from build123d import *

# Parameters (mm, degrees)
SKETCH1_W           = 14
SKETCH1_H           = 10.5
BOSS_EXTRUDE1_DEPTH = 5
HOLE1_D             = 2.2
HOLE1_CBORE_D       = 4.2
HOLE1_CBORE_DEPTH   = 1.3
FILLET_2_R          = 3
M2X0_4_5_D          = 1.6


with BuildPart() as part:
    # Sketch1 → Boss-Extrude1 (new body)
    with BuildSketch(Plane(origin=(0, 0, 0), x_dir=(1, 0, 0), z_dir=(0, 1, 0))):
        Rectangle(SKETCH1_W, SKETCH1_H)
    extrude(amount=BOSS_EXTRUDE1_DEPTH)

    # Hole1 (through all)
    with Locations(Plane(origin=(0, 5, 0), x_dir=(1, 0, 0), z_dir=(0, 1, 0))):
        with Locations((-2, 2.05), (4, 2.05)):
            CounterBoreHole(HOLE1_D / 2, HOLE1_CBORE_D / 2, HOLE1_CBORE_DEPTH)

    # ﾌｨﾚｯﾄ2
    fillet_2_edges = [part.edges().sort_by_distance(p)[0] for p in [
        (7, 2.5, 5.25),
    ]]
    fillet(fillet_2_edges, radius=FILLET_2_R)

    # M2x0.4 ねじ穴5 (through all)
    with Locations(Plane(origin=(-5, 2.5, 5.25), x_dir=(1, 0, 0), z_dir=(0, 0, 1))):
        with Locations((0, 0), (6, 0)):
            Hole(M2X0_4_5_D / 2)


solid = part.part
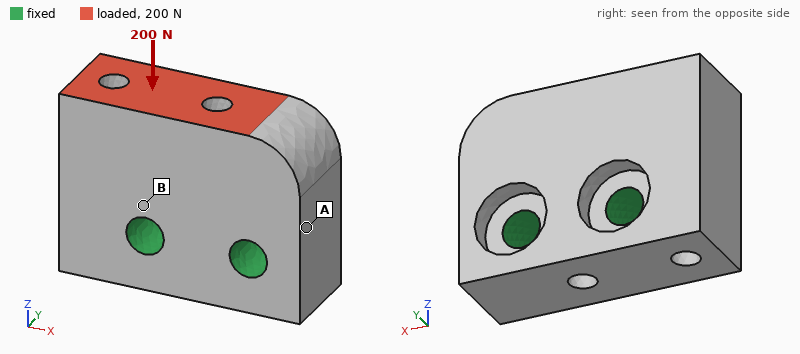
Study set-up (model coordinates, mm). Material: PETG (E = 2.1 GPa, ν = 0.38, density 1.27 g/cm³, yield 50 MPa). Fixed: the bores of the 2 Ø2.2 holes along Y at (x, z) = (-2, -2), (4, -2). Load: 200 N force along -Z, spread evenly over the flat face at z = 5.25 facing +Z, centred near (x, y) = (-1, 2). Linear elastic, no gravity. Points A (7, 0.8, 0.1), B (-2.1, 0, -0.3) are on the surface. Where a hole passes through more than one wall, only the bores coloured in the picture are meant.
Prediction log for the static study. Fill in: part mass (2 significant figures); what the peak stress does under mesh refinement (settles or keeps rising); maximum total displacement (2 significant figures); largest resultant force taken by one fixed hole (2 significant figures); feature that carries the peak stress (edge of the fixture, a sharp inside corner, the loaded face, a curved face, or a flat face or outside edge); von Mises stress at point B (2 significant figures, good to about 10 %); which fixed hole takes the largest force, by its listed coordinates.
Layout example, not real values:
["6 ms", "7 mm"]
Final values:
["0.79 g", "keeps rising", "45 µm", "160 N", "edge of the fixture", "5.7 MPa", "(-2, -2)"]
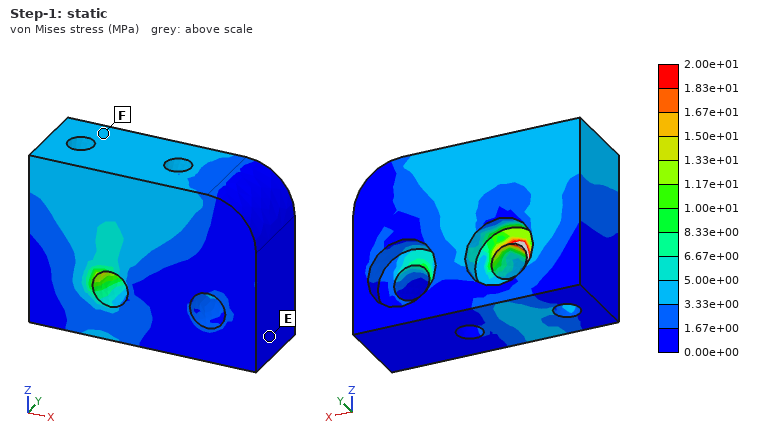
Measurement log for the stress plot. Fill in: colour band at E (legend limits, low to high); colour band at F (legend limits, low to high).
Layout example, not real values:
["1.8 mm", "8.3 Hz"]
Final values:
["0.00e+00 to 1.67e+00 MPa", "3.33e+00 to 5.00e+00 MPa"]
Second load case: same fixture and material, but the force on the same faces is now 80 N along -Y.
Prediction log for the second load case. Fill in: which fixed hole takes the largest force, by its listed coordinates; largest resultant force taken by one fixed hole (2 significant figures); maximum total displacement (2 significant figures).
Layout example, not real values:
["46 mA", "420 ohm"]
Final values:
["(-2, -2)", "60 N", "0.11 mm"]
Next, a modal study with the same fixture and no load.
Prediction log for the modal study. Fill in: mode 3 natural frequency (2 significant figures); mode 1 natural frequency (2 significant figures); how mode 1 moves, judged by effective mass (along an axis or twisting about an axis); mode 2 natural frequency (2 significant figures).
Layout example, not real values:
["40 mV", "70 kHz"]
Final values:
["16 kHz", "12 kHz", "along Y", "16 kHz"]
